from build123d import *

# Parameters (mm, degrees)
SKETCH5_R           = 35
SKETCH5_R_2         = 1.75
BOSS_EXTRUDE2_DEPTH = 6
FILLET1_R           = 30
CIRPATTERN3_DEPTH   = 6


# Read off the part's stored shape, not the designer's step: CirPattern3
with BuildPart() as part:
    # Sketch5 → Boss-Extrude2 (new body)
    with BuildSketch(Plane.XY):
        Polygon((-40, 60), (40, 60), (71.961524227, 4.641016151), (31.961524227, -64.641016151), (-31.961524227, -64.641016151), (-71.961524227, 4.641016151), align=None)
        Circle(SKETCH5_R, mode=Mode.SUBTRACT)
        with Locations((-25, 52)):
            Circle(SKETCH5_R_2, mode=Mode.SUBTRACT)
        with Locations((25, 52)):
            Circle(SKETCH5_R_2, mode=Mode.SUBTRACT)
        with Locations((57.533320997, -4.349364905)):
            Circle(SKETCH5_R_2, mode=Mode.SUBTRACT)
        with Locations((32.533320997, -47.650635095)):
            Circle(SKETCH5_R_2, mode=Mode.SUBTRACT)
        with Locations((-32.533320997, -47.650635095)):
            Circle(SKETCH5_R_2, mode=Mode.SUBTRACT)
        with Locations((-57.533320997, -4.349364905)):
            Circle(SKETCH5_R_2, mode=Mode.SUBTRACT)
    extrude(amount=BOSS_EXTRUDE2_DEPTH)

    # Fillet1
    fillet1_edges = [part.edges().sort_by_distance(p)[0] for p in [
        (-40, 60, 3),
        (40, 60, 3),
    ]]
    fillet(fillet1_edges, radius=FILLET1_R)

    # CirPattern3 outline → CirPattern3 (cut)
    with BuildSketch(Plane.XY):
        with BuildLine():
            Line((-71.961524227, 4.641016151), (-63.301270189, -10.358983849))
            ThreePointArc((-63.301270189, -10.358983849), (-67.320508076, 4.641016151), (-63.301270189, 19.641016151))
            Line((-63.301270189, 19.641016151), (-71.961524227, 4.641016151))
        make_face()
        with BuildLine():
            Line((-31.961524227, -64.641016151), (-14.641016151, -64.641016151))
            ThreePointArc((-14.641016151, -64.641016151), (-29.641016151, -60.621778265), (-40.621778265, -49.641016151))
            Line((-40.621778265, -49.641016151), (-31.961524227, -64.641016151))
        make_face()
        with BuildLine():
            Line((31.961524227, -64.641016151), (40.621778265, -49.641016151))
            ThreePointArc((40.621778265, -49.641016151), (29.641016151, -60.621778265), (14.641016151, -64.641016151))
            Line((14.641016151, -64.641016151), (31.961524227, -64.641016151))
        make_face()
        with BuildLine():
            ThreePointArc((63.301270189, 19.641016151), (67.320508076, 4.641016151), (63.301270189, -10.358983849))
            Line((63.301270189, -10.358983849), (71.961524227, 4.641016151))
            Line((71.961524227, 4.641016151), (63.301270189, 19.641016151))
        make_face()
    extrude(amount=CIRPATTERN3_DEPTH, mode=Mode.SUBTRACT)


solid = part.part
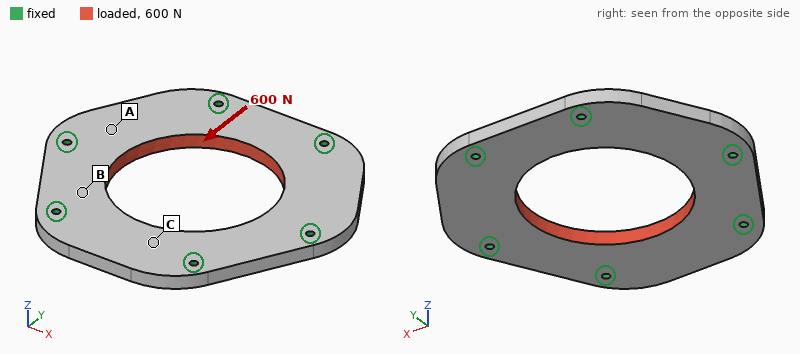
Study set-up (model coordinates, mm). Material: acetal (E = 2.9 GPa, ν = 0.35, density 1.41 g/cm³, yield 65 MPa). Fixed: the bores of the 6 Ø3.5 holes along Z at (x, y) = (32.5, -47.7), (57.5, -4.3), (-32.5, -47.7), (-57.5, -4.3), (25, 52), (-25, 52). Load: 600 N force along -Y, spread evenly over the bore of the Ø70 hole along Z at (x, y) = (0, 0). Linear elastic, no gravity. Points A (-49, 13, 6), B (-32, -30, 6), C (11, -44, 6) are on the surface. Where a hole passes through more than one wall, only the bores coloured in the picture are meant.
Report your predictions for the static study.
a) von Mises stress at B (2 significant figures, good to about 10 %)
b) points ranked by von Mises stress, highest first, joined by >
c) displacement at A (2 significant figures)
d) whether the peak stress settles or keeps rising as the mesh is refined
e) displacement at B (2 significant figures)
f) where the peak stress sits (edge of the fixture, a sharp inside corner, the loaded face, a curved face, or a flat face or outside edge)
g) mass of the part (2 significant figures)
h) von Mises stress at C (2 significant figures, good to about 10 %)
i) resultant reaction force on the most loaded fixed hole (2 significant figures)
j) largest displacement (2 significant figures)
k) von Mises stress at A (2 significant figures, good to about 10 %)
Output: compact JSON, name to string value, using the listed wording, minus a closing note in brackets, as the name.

{"von Mises stress at B": "0.86 MPa", "points ranked by von Mises stress, highest first, joined by >": "B > C > A", "displacement at A": "6.0 µm", "whether the peak stress settles or keeps rising as the mesh is refined": "keeps rising", "displacement at B": "5.9 µm", "where the peak stress sits": "edge of the fixture", "mass of the part": "78 g", "von Mises stress at C": "0.45 MPa", "resultant reaction force on the most loaded fixed hole": "120 N", "largest displacement": "15 µm", "von Mises stress at A": "0.30 MPa"}
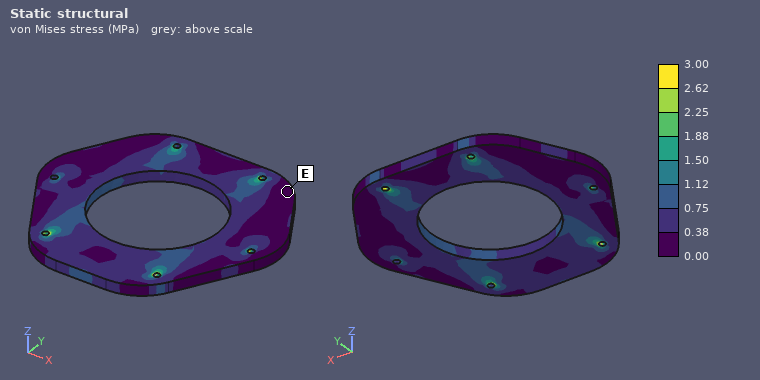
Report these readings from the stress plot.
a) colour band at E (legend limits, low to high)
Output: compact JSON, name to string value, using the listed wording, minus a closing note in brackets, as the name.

{"colour band at E": "0.00 to 0.38 MPa"}
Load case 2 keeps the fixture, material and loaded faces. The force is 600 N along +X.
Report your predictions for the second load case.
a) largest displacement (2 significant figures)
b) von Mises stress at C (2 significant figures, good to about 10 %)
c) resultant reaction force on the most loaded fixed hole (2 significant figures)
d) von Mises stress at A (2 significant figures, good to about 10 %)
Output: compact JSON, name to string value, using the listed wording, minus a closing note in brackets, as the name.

{"largest displacement": "13 µm", "von Mises stress at C": "0.50 MPa", "resultant reaction force on the most loaded fixed hole": "130 N", "von Mises stress at A": "0.51 MPa"}
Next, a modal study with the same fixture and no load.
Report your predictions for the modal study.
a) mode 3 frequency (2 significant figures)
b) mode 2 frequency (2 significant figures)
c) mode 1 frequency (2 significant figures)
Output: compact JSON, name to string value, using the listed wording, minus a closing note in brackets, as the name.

{"mode 3 frequency": "1700 Hz", "mode 2 frequency": "1700 Hz", "mode 1 frequency": "1700 Hz"}
